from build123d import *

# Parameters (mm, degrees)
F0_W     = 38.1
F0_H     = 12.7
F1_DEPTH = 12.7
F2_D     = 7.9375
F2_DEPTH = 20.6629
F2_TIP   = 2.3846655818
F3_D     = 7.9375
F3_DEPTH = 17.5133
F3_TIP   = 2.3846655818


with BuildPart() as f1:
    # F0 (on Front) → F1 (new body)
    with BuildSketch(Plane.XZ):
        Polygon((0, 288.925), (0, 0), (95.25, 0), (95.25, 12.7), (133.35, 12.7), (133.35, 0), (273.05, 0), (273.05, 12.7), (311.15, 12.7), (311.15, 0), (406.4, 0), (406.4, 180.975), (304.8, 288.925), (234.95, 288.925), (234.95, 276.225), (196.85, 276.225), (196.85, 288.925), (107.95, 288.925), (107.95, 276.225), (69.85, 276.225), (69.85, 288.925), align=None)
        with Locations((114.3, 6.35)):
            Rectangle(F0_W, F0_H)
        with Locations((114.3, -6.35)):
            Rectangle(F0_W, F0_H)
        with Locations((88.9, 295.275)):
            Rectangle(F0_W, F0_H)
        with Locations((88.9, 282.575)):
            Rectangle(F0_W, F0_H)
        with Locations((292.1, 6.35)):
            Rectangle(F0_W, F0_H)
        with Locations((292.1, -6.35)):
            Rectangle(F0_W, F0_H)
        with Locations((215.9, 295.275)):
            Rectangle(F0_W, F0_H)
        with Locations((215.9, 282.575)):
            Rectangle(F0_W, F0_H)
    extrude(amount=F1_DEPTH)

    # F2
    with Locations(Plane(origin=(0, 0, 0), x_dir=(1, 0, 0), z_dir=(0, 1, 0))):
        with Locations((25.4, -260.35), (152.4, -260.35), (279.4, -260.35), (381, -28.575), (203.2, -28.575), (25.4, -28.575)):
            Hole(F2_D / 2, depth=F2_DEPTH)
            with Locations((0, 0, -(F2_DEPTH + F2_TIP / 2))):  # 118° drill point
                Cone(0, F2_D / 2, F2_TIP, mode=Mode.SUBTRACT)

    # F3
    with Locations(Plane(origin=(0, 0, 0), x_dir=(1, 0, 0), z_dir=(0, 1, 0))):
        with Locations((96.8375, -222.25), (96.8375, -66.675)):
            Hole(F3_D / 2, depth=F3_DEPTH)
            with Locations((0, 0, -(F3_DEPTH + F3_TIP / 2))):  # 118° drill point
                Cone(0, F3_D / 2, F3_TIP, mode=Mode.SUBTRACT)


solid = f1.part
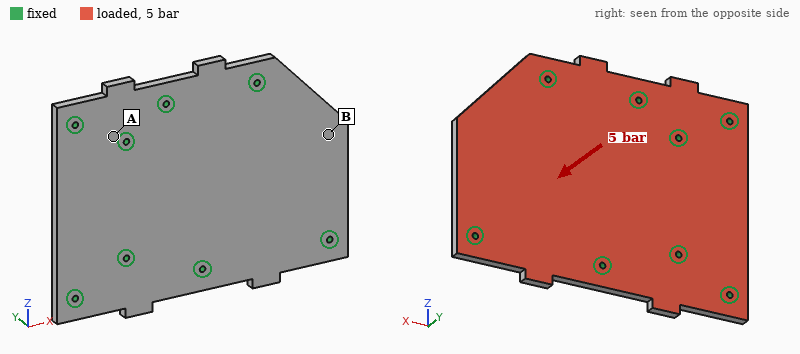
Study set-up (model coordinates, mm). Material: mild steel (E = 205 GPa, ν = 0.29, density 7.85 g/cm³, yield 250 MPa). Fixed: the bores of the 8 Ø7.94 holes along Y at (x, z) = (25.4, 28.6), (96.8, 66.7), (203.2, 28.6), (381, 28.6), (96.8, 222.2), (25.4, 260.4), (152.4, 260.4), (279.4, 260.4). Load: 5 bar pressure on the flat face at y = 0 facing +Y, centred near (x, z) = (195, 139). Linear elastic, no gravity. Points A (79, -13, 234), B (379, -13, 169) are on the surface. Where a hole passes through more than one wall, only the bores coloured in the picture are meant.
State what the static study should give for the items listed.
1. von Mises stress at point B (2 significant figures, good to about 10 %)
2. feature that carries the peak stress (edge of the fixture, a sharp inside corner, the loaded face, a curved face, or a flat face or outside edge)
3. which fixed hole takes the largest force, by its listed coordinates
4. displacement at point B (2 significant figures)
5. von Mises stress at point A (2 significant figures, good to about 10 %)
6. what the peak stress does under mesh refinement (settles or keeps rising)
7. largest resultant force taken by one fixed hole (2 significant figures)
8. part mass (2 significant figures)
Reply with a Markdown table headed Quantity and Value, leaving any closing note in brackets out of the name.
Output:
| Quantity | Value |
|---|---|
| von Mises stress at point B | 56 MPa |
| feature that carries the peak stress | edge of the fixture |
| which fixed hole takes the largest force, by its listed coordinates | (279.4, 260.4) |
| displacement at point B | 0.29 mm |
| von Mises stress at point A | 23 MPa |
| what the peak stress does under mesh refinement | keeps rising |
| largest resultant force taken by one fixed hole | 12 kN |
| part mass | 11 kg |
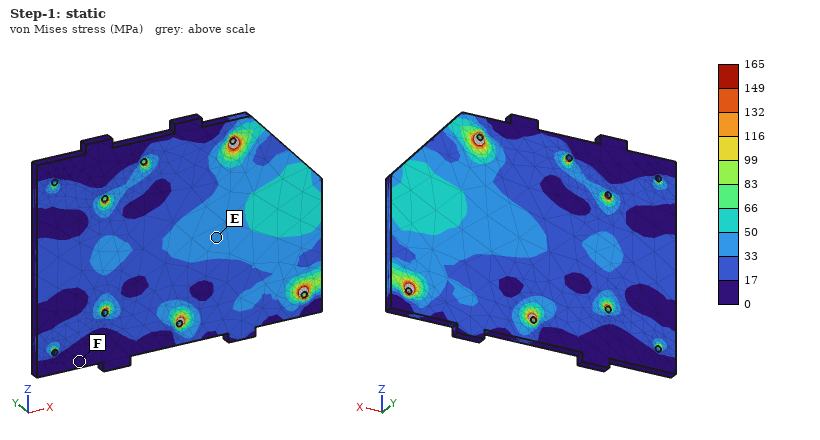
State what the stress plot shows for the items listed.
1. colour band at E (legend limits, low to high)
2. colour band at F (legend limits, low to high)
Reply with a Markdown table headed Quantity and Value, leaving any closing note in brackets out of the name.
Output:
| Quantity | Value |
|---|---|
| colour band at E | 33 to 50 MPa |
| colour band at F | 0 to 17 MPa |
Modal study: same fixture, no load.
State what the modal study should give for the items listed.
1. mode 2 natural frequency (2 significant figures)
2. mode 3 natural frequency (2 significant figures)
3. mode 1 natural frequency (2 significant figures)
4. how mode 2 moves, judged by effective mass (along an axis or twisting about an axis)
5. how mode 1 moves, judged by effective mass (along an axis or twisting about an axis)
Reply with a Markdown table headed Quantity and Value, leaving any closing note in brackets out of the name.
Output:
| Quantity | Value |
|---|---|
| mode 2 natural frequency | 1200 Hz |
| mode 3 natural frequency | 1500 Hz |
| mode 1 natural frequency | 800 Hz |
| how mode 2 moves, judged by effective mass | along Y |
| how mode 1 moves, judged by effective mass | along Y |
